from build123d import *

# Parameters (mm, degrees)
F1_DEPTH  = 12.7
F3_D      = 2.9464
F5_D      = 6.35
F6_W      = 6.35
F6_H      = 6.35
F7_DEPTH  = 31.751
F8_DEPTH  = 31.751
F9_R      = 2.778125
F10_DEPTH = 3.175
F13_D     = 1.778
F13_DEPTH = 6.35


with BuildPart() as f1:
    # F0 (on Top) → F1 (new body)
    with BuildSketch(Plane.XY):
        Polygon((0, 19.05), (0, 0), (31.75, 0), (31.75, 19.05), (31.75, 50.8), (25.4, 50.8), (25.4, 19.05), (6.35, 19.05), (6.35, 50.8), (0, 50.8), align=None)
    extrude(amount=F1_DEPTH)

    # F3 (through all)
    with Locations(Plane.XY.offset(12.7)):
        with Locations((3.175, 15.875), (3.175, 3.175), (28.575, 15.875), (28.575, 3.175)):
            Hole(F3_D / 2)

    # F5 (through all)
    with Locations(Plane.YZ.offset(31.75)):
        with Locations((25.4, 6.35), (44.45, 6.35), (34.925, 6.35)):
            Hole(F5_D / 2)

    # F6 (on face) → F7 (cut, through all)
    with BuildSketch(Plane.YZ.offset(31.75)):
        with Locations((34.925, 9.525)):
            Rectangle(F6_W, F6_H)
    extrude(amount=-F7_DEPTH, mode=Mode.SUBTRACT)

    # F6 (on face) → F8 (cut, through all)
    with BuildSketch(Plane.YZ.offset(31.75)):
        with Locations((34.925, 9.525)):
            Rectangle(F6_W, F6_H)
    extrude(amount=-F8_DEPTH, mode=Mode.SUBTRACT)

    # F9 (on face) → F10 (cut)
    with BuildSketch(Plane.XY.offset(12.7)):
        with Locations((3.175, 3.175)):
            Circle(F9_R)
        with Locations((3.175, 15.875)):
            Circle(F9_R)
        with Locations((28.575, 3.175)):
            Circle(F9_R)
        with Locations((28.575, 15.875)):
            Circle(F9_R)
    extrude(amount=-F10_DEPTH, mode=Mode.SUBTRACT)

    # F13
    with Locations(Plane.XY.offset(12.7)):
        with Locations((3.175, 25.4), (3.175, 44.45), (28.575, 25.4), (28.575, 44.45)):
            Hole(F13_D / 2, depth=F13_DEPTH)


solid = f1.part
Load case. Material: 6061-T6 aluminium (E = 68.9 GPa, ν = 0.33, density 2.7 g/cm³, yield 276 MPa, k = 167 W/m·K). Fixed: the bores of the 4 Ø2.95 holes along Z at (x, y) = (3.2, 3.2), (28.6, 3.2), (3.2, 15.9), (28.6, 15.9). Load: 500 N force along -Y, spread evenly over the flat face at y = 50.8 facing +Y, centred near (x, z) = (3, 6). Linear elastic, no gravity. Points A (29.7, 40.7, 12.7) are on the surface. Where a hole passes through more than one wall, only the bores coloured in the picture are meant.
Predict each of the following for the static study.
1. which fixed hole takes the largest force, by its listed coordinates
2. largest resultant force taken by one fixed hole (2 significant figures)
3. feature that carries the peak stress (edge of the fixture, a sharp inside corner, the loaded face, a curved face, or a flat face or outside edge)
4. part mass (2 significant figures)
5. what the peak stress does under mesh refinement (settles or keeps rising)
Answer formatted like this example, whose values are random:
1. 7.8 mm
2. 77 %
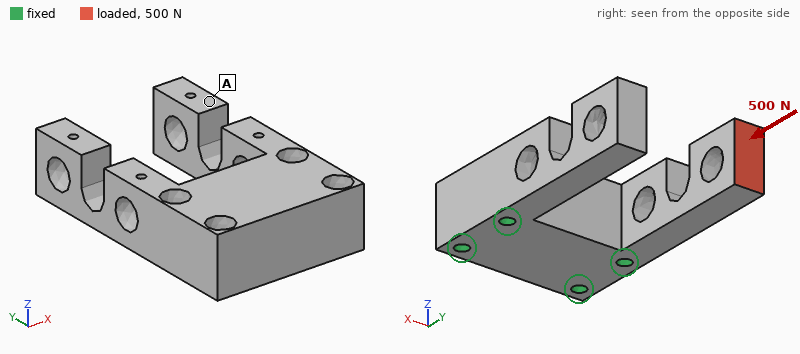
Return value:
1. (3.2, 15.9)
2. 440 N
3. a sharp inside corner
4. 29 g
5. keeps rising
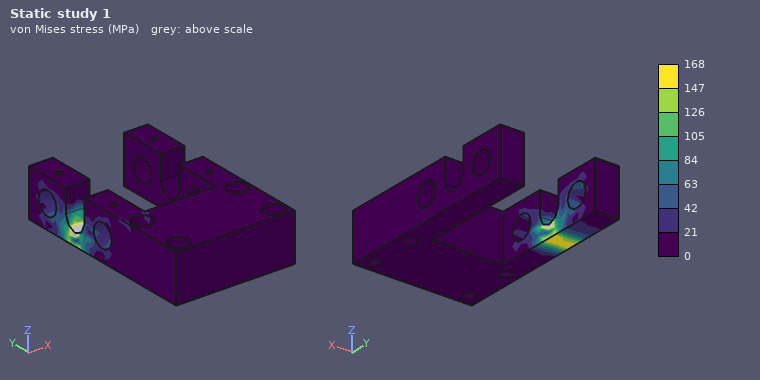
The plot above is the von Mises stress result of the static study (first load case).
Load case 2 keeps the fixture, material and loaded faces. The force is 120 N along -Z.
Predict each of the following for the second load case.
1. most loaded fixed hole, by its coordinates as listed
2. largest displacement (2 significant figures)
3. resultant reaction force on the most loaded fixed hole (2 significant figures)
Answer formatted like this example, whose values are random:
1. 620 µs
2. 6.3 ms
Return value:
1. (3.2, 15.9)
2. 0.25 mm
3. 210 N
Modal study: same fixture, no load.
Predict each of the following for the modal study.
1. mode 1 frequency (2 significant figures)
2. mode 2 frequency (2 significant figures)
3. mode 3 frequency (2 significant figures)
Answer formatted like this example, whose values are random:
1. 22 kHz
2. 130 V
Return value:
1. 3300 Hz
2. 3300 Hz
3. 3400 Hz
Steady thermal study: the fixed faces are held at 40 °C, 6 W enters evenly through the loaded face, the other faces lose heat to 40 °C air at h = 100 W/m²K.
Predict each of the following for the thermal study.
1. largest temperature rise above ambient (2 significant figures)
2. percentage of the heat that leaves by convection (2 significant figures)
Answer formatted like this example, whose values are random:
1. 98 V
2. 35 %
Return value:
1. 27 K
2. 30 %
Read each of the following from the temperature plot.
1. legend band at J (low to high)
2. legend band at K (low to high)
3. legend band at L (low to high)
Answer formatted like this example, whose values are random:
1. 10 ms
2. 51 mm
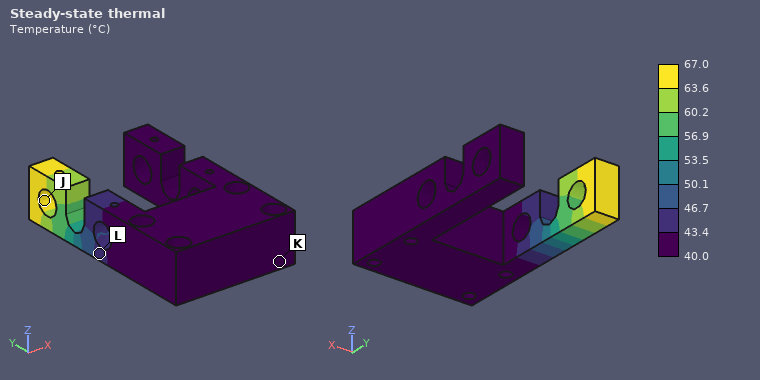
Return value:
1. 63.6 to 67.0 °C
2. 40.0 to 43.4 °C
3. 43.4 to 46.7 °C
